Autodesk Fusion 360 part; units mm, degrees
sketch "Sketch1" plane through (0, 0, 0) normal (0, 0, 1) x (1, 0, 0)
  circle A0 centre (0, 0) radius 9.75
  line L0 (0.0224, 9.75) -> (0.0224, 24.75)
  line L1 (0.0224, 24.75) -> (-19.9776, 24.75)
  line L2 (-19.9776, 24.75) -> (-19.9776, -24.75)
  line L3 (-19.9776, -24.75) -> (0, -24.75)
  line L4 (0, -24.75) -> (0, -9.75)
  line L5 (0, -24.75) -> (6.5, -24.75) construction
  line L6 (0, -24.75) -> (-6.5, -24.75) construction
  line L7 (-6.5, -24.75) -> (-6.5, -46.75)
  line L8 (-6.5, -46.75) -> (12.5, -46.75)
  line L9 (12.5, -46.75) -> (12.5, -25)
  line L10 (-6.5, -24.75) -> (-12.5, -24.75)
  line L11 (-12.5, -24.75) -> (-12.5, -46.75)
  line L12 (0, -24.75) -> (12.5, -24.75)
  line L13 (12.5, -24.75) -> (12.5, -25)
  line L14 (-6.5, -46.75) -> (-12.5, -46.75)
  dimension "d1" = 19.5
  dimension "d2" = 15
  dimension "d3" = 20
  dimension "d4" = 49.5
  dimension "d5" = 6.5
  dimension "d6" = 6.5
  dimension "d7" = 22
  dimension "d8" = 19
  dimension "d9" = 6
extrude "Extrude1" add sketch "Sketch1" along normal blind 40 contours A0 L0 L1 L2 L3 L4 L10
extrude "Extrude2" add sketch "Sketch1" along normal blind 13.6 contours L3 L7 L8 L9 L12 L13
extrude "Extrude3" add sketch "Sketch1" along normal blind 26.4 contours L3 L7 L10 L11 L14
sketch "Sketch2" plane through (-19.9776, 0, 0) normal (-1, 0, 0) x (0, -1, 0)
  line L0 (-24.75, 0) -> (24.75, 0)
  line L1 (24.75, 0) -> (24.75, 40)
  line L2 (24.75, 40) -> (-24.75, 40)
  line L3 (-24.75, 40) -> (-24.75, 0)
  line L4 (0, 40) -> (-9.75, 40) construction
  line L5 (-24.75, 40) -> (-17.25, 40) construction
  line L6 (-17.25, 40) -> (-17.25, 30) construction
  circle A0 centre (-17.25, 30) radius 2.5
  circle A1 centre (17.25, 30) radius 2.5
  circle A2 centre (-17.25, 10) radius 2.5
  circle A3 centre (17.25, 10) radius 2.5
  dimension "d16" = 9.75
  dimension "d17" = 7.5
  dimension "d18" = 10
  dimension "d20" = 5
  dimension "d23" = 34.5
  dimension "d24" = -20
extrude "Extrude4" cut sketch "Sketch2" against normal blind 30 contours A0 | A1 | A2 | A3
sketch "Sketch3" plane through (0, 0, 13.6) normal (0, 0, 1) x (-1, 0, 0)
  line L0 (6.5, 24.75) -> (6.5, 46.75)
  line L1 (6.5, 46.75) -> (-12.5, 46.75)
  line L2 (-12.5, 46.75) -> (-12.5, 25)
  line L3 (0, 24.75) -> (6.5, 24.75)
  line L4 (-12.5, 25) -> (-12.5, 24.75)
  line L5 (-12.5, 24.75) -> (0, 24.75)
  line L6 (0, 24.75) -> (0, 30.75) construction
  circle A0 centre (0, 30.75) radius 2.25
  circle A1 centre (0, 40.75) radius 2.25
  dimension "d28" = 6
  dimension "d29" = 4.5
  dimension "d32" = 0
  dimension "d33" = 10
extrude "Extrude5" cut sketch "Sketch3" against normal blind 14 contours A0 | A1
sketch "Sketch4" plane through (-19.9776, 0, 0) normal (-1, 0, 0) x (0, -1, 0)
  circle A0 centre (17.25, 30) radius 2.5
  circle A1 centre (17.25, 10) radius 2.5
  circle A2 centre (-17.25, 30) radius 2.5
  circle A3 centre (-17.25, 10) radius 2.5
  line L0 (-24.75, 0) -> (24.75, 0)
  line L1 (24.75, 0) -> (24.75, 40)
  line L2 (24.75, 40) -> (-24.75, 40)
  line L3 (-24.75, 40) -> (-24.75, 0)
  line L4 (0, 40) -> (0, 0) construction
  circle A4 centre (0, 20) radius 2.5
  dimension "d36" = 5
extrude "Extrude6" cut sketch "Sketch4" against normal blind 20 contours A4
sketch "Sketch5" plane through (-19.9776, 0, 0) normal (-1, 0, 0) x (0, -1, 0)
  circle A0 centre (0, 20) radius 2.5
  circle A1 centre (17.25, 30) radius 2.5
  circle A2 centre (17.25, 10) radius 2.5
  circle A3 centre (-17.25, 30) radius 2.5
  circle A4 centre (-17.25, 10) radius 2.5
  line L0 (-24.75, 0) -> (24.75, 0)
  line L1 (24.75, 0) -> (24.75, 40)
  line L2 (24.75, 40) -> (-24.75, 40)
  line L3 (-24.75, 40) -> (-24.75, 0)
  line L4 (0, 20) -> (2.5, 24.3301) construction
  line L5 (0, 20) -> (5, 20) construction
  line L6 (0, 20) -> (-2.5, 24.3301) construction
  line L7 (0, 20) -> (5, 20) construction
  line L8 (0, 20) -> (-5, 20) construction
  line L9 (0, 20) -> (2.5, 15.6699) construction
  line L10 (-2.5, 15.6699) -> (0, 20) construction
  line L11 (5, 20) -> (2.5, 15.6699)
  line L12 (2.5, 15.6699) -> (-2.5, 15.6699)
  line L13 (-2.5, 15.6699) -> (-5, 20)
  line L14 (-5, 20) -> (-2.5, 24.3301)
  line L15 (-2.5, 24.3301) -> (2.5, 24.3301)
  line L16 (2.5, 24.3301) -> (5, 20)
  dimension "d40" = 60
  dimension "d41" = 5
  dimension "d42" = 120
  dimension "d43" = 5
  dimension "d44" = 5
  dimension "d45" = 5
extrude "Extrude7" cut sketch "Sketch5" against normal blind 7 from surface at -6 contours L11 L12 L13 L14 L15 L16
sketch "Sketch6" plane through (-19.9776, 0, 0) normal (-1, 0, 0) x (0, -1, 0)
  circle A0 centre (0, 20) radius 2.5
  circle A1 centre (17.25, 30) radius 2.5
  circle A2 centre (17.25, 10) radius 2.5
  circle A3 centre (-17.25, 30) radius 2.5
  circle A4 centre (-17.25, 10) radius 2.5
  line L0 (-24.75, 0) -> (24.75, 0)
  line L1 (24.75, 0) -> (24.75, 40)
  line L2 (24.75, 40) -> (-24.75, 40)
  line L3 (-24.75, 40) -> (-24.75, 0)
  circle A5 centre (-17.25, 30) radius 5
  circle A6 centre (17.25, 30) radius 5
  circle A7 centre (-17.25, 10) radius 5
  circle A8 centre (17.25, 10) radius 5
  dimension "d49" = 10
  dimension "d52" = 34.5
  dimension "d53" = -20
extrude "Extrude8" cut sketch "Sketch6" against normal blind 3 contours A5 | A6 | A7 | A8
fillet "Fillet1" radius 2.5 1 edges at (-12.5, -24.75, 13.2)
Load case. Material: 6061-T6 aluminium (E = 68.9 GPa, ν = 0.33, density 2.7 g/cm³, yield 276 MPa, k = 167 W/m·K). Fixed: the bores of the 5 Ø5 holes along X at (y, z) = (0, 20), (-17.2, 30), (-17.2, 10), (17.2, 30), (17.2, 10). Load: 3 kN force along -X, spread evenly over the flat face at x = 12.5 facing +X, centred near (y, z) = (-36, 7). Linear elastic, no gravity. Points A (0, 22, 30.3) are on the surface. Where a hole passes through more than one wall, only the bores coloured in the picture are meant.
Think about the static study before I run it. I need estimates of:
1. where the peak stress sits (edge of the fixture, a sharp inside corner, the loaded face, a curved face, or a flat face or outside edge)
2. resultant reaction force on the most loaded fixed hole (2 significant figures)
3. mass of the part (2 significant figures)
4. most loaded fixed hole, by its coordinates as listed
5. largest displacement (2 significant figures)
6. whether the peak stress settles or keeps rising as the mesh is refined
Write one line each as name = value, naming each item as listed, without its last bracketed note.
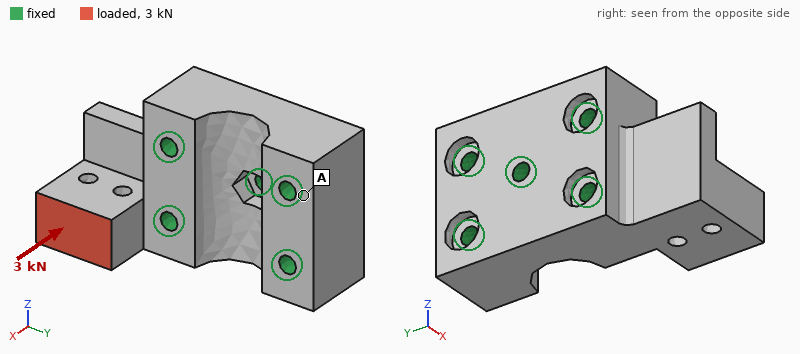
where the peak stress sits = edge of the fixture
resultant reaction force on the most loaded fixed hole = 3.1 kN
mass of the part = 110 g
most loaded fixed hole, by its coordinates as listed = (-17.2, 10)
largest displacement = 68 µm
whether the peak stress settles or keeps rising as the mesh is refined = keeps rising
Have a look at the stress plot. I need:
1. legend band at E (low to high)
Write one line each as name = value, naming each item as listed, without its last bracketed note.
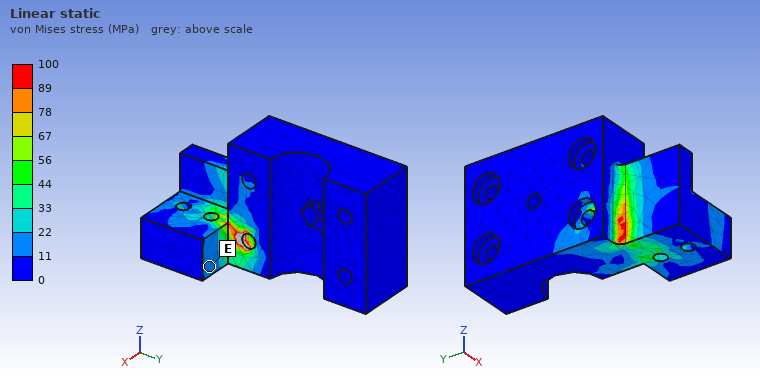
legend band at E = 11 to 22 MPa
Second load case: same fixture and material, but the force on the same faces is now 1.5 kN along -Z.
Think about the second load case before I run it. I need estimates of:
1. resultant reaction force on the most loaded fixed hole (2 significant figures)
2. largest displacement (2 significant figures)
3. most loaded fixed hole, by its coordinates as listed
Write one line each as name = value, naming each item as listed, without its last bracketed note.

resultant reaction force on the most loaded fixed hole = 1.4 kN
largest displacement = 64 µm
most loaded fixed hole, by its coordinates as listed = (-17.2, 10)
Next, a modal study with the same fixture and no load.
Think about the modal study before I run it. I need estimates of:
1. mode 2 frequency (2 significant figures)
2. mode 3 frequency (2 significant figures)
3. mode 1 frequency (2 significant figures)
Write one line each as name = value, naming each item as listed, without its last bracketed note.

mode 2 frequency = 10 kHz
mode 3 frequency = 17 kHz
mode 1 frequency = 8300 Hz
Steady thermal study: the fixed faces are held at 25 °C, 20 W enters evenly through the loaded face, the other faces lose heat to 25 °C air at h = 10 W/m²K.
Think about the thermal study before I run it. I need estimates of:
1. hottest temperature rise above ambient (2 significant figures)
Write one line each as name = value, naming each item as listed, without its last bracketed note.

hottest temperature rise above ambient = 14 K
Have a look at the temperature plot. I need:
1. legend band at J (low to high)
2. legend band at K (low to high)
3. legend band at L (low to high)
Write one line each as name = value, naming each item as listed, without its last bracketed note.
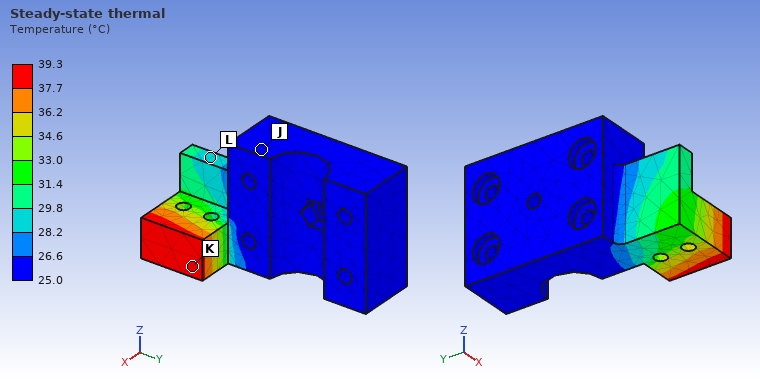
legend band at J = 25.0 to 26.6 °C
legend band at K = 37.7 to 39.3 °C
legend band at L = 28.2 to 29.8 °C
